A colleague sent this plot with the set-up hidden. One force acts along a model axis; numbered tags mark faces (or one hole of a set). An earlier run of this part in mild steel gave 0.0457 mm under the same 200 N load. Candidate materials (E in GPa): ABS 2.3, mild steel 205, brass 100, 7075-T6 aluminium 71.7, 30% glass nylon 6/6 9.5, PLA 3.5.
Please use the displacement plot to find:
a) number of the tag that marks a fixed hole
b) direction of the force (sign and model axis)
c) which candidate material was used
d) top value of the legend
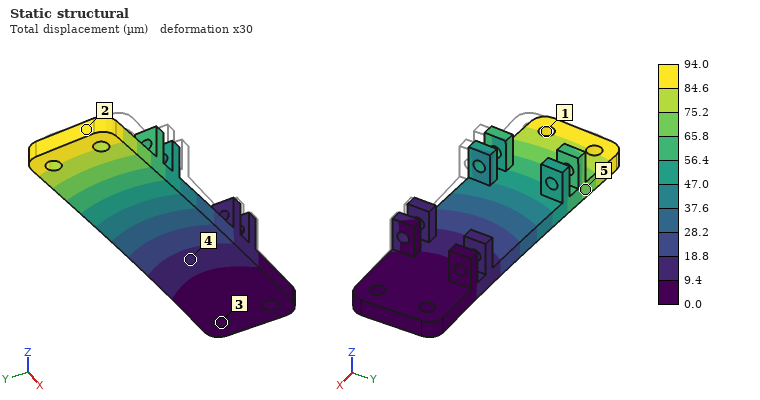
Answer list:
3
+Y
brass
94.0 µm
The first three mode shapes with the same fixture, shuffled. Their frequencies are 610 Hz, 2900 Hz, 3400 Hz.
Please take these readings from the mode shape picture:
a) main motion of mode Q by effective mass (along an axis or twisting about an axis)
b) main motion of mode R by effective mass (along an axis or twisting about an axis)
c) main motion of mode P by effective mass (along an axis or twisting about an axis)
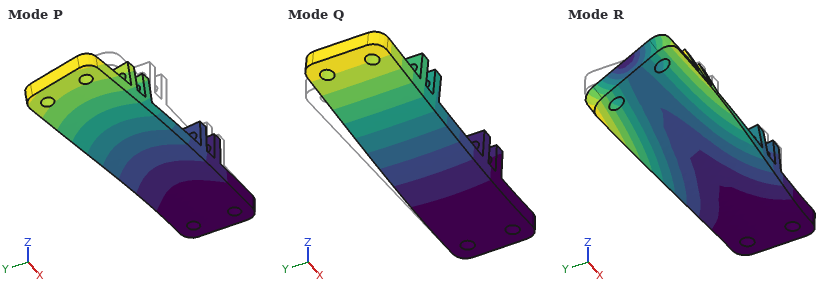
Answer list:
along Z
twisting about X
along Y
